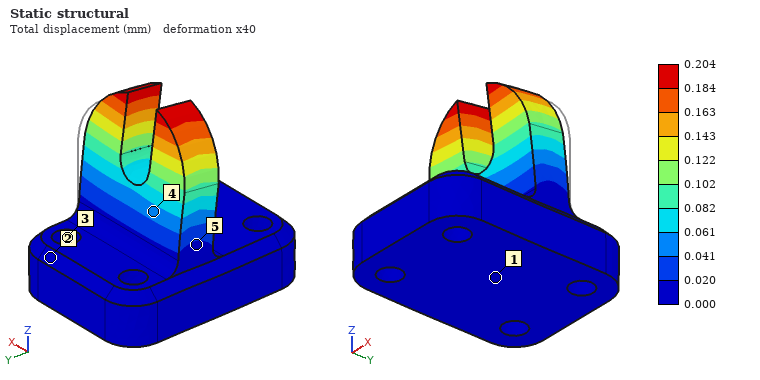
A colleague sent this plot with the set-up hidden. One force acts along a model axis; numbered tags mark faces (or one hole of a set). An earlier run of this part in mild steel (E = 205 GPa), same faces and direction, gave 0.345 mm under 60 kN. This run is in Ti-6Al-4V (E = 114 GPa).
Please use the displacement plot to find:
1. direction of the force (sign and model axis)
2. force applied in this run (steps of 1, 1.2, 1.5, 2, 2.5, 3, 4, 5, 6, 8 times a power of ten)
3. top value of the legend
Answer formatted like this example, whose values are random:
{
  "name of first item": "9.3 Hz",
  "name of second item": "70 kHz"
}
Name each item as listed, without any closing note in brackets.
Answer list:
{
  "direction of the force": "-Y",
  "force applied in this run": "20 kN",
  "top value of the legend": "0.204 mm"
}
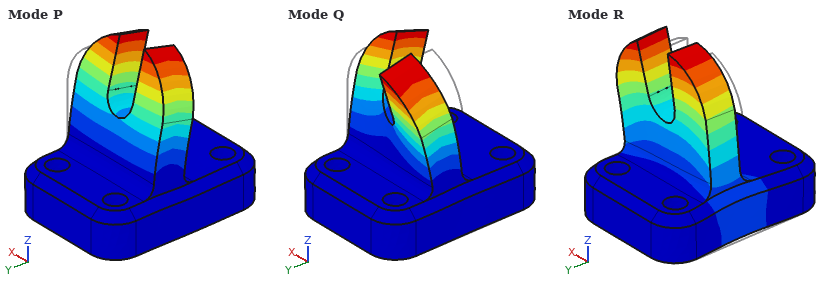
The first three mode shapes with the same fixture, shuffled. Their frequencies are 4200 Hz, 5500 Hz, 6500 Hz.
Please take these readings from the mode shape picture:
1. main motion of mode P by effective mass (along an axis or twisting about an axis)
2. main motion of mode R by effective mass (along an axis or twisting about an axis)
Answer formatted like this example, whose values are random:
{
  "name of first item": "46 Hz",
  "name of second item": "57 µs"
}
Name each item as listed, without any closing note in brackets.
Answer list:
{
  "main motion of mode P by effective mass": "along Y",
  "main motion of mode R by effective mass": "along X"
}
